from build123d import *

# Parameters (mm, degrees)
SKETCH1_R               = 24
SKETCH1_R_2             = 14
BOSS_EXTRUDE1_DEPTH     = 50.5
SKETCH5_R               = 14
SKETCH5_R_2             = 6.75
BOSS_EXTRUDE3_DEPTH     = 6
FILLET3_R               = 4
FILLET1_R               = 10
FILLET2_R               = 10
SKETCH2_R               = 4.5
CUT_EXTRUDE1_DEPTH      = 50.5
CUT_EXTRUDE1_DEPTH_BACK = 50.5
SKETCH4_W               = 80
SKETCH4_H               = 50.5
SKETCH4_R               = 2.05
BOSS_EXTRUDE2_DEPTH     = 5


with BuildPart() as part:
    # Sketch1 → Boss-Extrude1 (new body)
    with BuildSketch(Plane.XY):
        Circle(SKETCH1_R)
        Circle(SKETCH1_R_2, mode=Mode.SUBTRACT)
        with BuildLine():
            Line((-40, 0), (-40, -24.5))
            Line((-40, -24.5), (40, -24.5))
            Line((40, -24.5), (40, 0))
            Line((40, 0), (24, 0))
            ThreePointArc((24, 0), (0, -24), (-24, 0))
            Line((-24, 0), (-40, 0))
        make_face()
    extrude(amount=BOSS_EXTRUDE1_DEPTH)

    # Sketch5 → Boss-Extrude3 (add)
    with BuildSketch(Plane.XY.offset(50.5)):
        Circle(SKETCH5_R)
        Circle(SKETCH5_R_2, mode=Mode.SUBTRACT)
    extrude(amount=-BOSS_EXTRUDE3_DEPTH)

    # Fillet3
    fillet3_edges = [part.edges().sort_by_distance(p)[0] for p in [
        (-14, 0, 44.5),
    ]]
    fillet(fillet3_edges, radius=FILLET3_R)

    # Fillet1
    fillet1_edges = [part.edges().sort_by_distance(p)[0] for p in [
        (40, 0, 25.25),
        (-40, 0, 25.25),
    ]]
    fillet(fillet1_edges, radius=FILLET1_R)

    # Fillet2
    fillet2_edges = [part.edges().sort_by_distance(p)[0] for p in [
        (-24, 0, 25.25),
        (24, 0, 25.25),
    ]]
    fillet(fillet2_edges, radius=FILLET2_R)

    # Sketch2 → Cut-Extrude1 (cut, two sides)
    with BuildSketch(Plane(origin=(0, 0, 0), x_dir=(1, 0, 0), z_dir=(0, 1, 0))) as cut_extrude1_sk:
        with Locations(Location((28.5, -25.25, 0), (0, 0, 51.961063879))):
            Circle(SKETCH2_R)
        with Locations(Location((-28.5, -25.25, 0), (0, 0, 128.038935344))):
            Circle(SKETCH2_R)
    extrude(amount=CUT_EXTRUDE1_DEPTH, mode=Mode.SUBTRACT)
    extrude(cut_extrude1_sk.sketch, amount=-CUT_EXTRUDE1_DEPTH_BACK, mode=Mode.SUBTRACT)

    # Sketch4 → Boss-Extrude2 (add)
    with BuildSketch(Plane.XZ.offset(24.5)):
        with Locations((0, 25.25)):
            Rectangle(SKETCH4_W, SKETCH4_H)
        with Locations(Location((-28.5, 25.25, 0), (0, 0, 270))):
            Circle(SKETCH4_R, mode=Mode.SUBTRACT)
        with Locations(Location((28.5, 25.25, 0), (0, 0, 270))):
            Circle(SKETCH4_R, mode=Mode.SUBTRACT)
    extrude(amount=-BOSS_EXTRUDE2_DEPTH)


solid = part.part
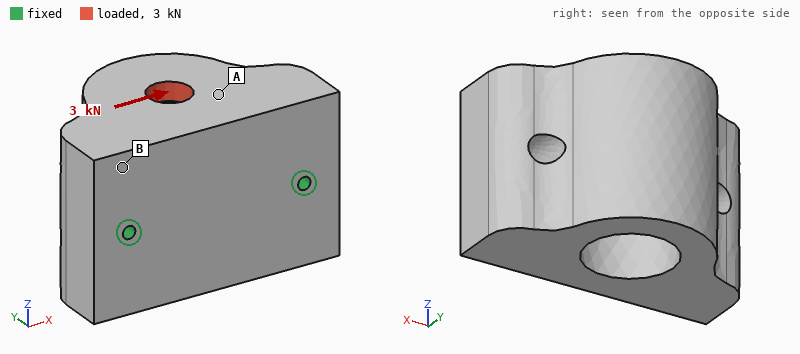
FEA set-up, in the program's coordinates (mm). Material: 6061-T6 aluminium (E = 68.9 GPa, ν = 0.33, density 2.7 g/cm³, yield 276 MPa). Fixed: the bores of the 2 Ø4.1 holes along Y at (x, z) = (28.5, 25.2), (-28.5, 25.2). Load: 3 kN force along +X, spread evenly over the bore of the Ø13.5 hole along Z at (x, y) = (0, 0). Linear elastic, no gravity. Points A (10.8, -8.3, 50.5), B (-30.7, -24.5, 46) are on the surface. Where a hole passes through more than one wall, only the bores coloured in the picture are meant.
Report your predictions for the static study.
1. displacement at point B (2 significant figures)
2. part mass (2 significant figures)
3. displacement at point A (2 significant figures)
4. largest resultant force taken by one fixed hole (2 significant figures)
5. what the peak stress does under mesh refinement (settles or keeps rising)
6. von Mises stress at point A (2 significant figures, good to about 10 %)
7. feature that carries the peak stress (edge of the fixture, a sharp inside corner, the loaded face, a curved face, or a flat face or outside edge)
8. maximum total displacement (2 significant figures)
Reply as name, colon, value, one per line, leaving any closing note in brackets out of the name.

displacement at point B: 5.3 µm
part mass: 310 g
displacement at point A: 7.7 µm
largest resultant force taken by one fixed hole: 2.2 kN
what the peak stress does under mesh refinement: keeps rising
von Mises stress at point A: 10 MPa
feature that carries the peak stress: edge of the fixture
maximum total displacement: 12 µm
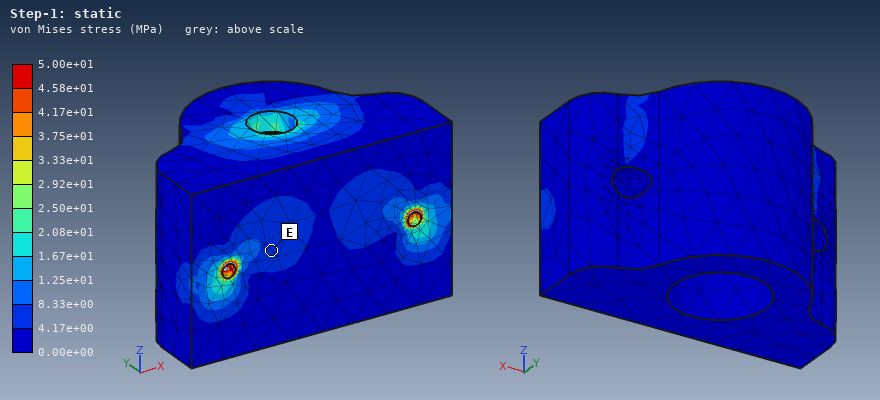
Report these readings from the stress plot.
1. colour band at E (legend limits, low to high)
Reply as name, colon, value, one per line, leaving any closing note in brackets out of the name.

colour band at E: 4.17e+00 to 8.33e+00 MPa
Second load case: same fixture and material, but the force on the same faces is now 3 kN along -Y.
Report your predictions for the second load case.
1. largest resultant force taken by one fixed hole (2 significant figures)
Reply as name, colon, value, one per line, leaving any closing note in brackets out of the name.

largest resultant force taken by one fixed hole: 1.6 kN
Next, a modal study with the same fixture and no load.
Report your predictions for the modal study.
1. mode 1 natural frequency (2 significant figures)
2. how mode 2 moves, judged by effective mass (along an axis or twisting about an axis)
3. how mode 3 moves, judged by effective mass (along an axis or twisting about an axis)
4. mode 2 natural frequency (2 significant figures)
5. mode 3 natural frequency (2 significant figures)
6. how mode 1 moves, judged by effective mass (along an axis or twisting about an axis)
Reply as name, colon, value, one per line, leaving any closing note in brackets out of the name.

mode 1 natural frequency: 1300 Hz
how mode 2 moves, judged by effective mass: along X
how mode 3 moves, judged by effective mass: along Y
mode 2 natural frequency: 6600 Hz
mode 3 natural frequency: 7800 Hz
how mode 1 moves, judged by effective mass: along Z
